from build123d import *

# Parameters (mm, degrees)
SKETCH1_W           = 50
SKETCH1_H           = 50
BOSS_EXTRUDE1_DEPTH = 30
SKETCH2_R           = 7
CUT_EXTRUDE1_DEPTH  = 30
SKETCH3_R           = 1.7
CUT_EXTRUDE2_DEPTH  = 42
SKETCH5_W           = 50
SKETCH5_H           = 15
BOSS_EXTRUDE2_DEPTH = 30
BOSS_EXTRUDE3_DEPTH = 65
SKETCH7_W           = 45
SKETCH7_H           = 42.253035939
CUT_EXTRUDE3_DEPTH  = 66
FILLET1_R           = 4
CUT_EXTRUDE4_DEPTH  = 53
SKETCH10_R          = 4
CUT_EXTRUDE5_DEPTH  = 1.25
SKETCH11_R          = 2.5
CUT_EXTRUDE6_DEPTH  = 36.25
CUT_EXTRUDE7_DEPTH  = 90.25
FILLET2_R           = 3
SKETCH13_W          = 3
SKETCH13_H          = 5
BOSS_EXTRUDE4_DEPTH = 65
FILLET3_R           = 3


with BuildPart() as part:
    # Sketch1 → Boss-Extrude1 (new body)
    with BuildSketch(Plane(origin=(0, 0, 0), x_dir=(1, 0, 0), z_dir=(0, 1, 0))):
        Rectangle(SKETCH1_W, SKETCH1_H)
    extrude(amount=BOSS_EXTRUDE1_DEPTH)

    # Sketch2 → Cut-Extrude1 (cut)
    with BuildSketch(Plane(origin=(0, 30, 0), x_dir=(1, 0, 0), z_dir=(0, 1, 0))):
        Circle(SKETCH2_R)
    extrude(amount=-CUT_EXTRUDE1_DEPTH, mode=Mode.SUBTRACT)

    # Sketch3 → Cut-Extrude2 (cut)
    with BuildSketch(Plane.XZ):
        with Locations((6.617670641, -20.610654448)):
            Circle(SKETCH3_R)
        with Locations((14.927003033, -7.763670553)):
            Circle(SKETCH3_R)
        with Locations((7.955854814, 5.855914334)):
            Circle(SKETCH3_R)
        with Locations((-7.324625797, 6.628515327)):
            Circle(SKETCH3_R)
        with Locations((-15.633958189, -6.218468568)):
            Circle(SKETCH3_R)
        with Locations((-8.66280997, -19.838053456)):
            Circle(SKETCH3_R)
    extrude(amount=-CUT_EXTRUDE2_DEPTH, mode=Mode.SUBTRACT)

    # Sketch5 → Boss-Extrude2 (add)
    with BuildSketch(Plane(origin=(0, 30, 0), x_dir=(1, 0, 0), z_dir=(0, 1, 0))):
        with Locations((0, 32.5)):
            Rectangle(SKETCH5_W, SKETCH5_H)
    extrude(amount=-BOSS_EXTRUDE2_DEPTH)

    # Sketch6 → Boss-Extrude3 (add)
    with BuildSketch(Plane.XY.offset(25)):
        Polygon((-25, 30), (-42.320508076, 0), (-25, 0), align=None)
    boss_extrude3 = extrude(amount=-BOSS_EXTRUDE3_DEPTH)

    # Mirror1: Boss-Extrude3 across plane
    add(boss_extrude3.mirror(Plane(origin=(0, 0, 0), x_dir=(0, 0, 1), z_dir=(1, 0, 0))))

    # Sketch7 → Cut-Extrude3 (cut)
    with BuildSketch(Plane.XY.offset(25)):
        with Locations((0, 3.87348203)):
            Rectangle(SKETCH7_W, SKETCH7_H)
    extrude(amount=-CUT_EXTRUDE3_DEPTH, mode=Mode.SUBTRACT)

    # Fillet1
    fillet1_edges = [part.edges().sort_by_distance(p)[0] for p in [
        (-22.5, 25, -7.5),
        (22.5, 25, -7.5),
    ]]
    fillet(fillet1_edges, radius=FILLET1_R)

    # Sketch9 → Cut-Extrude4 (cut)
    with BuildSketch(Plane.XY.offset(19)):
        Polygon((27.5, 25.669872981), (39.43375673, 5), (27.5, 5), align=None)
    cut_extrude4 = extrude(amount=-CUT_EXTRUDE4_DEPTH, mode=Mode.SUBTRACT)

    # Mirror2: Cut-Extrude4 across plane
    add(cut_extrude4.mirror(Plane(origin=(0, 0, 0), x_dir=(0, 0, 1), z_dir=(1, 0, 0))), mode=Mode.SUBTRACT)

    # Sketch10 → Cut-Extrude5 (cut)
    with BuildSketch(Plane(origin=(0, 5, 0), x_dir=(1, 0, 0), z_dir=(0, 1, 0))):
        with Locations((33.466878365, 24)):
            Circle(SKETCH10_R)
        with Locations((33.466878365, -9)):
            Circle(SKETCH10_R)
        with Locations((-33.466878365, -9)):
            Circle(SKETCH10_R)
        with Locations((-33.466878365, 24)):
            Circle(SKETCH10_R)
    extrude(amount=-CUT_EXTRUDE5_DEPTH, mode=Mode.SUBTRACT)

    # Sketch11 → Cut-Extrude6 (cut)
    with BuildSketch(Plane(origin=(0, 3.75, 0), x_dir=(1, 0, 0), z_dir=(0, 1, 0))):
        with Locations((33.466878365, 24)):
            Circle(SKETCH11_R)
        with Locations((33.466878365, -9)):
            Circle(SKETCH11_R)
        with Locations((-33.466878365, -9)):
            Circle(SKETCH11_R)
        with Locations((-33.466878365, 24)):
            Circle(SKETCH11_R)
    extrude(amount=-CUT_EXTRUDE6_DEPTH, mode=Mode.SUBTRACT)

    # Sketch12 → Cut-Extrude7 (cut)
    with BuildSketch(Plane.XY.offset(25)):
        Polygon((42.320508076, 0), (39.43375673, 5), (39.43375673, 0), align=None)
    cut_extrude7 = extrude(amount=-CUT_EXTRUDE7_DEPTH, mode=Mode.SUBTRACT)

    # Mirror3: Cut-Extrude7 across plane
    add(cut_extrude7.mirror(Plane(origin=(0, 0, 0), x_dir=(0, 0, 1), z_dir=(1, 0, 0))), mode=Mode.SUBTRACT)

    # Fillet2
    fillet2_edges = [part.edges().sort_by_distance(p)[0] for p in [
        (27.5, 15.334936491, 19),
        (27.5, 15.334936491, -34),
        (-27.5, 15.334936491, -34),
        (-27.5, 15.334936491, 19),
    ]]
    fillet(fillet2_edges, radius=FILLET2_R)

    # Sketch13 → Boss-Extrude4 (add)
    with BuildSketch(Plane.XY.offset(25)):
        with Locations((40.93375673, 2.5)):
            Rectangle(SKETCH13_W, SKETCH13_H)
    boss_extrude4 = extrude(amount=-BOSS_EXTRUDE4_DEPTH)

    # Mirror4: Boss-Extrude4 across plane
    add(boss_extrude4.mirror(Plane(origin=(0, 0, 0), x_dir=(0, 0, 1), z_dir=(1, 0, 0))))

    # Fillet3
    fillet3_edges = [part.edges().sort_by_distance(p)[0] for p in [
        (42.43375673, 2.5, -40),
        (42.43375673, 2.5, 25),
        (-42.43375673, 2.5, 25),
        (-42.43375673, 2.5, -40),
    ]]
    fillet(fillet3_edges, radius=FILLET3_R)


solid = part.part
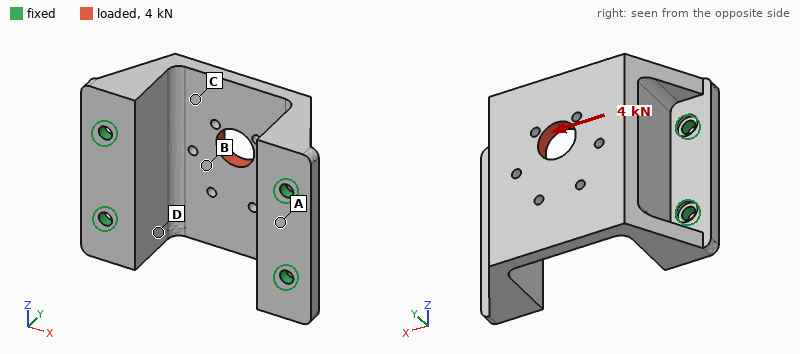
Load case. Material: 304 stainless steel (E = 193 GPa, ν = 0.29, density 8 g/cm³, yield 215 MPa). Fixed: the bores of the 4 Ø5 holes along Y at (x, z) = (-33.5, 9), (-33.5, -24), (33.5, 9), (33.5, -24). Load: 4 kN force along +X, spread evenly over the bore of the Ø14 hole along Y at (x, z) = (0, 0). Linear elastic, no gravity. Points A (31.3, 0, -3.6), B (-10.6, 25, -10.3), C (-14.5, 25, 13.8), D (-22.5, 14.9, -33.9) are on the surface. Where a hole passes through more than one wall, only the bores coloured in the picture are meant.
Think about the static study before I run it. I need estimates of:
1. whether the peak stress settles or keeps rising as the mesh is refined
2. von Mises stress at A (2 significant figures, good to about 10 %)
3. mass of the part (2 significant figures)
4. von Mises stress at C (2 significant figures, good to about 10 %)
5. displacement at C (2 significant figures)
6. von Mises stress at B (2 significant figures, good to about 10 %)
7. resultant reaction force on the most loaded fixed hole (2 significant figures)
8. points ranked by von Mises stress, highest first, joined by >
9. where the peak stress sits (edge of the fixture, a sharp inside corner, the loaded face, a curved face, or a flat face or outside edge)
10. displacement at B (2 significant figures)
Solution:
keeps rising
30 MPa
360 g
65 MPa
42 µm
48 MPa
1.3 kN
C > B > A > D
edge of the fixture
39 µm
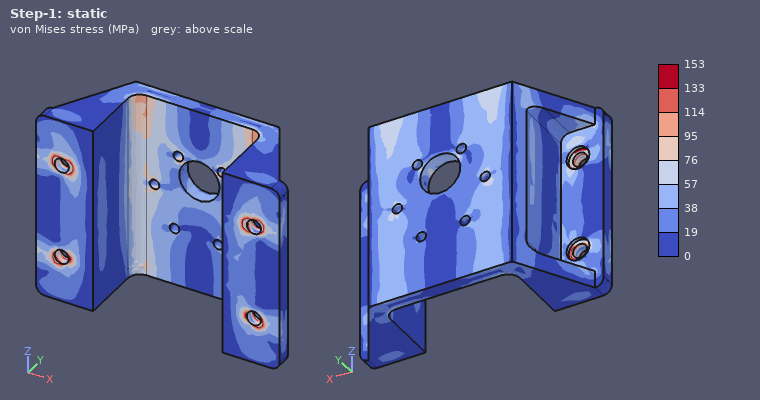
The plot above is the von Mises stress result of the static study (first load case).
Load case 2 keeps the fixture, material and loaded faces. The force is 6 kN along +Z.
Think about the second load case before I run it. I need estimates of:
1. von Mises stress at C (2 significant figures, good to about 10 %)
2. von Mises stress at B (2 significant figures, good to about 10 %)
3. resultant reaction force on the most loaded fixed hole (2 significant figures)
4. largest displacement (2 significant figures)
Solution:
21 MPa
23 MPa
2.8 kN
23 µm
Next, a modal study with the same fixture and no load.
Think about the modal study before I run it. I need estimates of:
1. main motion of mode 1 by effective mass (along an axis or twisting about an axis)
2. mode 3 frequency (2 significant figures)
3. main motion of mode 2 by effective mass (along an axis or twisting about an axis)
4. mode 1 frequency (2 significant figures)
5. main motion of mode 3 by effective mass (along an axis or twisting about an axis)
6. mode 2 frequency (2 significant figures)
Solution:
along X
6000 Hz
twisting about Y
3800 Hz
along Z
5700 Hz
